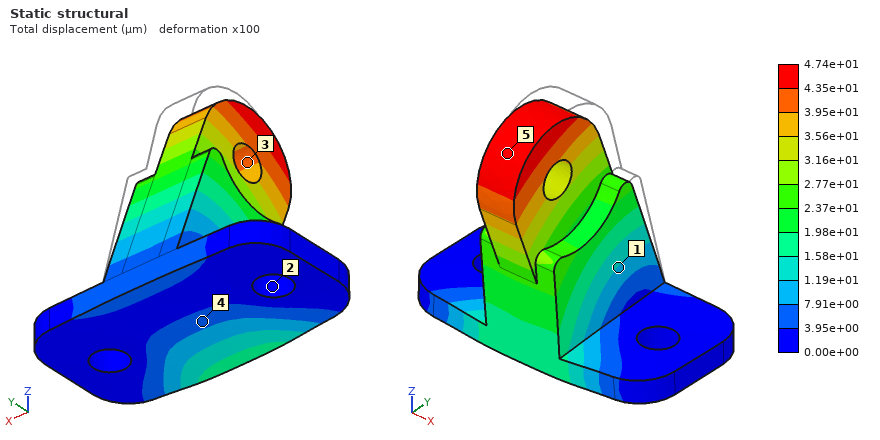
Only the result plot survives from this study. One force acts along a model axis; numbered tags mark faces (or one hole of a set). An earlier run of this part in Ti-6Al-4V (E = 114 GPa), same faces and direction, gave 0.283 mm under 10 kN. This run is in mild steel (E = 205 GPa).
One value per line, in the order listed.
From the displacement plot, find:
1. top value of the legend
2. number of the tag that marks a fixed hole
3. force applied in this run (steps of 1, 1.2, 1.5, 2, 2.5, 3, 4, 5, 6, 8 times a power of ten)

4.74e+01 µm
2
3 kN
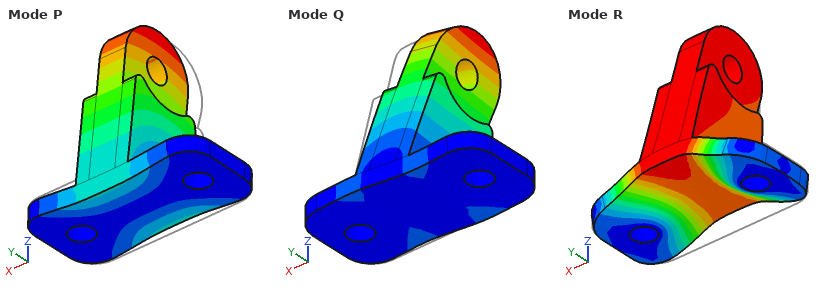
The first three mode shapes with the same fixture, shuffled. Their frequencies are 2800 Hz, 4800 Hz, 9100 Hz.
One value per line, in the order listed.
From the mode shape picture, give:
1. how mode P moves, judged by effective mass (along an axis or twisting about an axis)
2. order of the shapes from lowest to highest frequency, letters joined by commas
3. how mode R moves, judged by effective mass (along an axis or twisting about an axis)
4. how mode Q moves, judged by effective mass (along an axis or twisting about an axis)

along Y
P, Q, R
along Z
along X
